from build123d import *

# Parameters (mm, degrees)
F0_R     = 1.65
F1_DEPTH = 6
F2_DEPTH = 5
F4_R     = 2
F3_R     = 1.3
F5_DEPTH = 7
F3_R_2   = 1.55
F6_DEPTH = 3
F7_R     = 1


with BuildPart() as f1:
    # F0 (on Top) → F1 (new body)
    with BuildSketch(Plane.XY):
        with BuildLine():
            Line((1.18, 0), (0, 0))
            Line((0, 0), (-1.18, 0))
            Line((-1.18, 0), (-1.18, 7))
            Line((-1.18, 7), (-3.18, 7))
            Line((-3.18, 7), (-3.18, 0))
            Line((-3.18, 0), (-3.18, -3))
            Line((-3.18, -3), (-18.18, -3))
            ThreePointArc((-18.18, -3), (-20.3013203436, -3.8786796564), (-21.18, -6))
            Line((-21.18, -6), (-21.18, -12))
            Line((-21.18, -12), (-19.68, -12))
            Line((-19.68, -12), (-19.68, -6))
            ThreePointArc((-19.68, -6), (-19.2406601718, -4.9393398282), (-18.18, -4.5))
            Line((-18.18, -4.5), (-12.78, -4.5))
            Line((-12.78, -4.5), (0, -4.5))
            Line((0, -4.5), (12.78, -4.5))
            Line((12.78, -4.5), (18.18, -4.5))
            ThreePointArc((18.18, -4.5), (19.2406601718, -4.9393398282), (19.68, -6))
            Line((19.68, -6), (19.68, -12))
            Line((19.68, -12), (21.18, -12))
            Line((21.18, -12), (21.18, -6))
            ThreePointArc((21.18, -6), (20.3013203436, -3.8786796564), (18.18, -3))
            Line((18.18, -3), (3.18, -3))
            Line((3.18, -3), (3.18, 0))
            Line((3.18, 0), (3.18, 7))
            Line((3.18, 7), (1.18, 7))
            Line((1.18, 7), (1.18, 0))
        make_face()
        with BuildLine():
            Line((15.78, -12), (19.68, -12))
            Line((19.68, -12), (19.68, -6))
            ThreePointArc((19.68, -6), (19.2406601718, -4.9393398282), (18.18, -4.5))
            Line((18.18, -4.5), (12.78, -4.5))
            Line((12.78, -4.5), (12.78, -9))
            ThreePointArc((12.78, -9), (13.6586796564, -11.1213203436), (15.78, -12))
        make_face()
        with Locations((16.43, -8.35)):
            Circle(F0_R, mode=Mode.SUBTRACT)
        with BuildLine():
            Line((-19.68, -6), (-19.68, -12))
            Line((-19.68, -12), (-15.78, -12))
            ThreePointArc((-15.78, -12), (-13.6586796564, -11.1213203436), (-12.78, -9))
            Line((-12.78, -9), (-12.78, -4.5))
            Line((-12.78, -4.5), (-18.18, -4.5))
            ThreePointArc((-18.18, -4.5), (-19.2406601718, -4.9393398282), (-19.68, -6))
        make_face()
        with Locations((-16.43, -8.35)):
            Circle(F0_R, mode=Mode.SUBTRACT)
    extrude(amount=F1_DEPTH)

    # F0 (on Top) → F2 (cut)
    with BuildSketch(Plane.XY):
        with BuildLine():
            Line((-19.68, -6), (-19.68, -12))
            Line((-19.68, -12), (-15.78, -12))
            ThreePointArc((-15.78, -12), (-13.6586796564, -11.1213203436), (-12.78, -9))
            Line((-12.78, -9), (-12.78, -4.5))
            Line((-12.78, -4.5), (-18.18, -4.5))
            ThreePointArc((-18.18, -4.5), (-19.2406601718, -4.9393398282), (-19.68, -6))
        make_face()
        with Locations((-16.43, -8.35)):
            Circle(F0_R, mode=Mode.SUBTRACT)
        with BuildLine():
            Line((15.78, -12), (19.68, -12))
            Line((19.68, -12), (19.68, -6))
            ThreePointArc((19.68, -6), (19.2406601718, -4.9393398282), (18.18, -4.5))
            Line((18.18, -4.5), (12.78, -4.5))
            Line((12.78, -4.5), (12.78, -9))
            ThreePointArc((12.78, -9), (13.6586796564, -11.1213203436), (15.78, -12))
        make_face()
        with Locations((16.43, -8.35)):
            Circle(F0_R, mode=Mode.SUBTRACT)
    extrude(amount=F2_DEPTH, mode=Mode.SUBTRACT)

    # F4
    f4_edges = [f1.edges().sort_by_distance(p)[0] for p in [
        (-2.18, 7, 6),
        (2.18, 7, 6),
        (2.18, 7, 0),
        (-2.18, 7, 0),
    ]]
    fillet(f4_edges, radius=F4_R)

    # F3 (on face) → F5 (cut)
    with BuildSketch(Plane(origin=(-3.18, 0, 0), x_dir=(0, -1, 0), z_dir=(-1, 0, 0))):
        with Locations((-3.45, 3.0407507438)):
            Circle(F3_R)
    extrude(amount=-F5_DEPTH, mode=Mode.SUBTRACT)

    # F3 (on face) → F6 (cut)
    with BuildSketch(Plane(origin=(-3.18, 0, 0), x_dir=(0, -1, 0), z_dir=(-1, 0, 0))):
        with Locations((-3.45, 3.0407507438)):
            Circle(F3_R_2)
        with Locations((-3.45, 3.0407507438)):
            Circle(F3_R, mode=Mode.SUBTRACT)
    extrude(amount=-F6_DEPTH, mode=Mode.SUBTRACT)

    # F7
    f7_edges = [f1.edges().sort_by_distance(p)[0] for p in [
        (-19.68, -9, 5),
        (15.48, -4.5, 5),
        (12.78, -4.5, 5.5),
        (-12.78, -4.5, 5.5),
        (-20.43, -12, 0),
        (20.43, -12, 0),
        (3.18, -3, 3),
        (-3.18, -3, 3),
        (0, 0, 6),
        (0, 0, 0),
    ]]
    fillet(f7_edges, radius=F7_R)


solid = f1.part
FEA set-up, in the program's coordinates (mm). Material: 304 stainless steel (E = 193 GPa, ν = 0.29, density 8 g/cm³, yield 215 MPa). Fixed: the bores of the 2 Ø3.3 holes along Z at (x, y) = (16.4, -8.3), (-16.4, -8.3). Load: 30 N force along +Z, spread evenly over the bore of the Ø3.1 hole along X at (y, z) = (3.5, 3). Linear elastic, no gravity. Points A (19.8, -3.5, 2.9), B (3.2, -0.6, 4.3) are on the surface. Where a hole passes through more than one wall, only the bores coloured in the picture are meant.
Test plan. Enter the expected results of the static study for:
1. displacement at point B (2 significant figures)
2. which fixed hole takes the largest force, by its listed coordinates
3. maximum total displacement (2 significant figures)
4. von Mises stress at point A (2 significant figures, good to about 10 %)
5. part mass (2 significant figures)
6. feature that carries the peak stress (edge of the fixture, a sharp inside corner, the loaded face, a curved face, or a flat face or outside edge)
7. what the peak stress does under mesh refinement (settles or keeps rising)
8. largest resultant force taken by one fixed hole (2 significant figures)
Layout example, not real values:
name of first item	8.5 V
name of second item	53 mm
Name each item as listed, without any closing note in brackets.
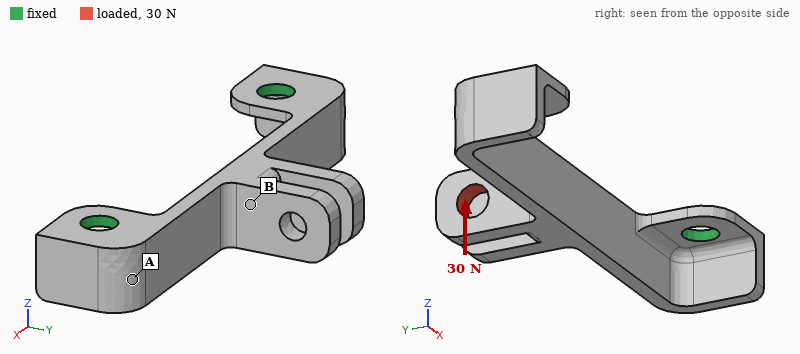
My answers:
displacement at point B	18 µm
which fixed hole takes the largest force, by its listed coordinates	(-16.4, -8.3)
maximum total displacement	51 µm
von Mises stress at point A	21 MPa
part mass	6.7 g
feature that carries the peak stress	edge of the fixture
what the peak stress does under mesh refinement	keeps rising
largest resultant force taken by one fixed hole	24 N
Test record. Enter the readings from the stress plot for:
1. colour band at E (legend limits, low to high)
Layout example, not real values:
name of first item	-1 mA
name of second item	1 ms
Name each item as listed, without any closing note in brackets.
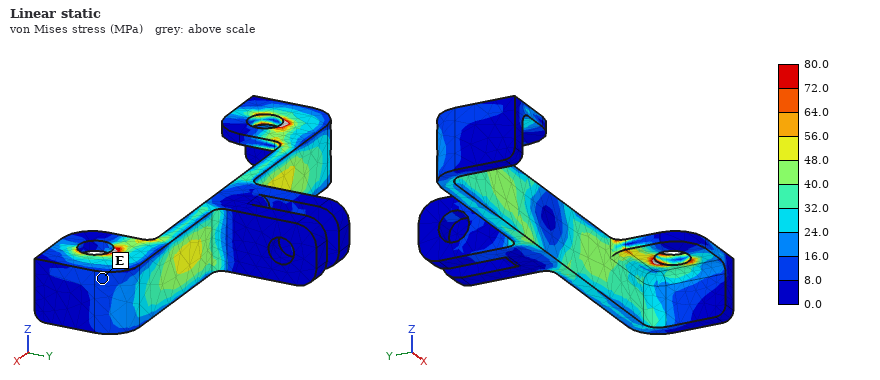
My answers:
colour band at E	8.0 to 16.0 MPa
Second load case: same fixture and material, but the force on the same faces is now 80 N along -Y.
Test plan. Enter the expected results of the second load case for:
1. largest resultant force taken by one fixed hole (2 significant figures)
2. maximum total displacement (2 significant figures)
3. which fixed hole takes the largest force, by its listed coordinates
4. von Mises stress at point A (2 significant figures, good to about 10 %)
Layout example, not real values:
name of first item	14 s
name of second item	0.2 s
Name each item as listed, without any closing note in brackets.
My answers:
largest resultant force taken by one fixed hole	61 N
maximum total displacement	37 µm
which fixed hole takes the largest force, by its listed coordinates	(-16.4, -8.3)
von Mises stress at point A	16 MPa
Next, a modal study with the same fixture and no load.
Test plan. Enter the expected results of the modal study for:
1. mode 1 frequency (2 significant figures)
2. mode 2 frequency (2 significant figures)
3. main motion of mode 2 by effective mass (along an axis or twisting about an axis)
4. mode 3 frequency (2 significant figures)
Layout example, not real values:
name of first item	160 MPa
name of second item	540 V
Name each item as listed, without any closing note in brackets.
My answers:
mode 1 frequency	3600 Hz
mode 2 frequency	6400 Hz
main motion of mode 2 by effective mass	along Y
mode 3 frequency	9900 Hz
